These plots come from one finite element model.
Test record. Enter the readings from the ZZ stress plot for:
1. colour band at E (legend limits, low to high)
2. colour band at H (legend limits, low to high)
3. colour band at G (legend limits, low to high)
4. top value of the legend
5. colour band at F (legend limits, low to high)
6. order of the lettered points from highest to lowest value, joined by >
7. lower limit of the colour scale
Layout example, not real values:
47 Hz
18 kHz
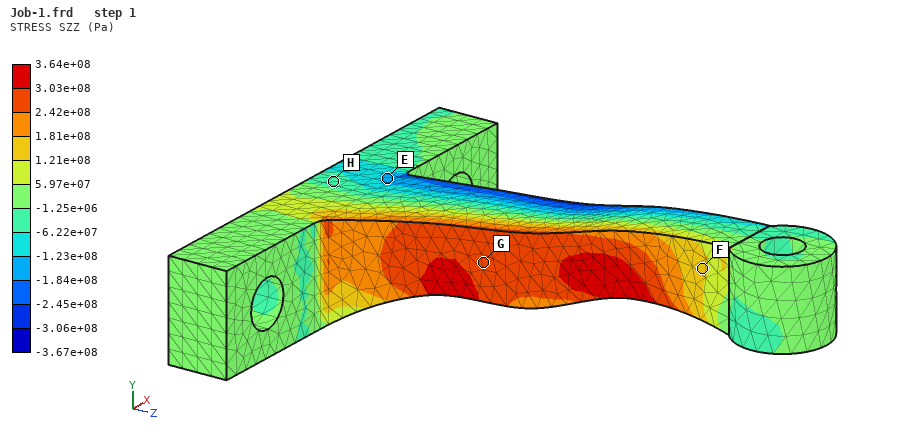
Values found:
-1.84e+08 to -1.23e+08 Pa
-6.22e+07 to -1.25e+06 Pa
2.42e+08 to 3.03e+08 Pa
3.64e+08 Pa
1.21e+08 to 1.81e+08 Pa
G > F > H > E
-3.67e+08 Pa
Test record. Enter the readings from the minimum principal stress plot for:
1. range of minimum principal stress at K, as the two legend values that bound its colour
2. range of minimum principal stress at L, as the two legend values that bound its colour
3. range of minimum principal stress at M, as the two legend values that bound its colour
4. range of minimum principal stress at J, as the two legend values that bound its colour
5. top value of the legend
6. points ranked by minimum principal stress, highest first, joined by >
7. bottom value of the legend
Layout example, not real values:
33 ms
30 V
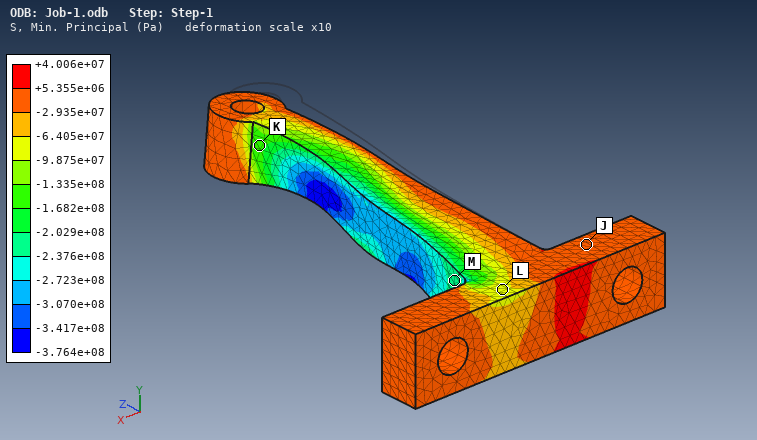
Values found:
-1.682e+08 to -1.335e+08 Pa
-9.875e+07 to -6.405e+07 Pa
-2.376e+08 to -2.029e+08 Pa
-2.935e+07 to +5.355e+06 Pa
+4.006e+07 Pa
J > L > K > M
-3.764e+08 Pa
